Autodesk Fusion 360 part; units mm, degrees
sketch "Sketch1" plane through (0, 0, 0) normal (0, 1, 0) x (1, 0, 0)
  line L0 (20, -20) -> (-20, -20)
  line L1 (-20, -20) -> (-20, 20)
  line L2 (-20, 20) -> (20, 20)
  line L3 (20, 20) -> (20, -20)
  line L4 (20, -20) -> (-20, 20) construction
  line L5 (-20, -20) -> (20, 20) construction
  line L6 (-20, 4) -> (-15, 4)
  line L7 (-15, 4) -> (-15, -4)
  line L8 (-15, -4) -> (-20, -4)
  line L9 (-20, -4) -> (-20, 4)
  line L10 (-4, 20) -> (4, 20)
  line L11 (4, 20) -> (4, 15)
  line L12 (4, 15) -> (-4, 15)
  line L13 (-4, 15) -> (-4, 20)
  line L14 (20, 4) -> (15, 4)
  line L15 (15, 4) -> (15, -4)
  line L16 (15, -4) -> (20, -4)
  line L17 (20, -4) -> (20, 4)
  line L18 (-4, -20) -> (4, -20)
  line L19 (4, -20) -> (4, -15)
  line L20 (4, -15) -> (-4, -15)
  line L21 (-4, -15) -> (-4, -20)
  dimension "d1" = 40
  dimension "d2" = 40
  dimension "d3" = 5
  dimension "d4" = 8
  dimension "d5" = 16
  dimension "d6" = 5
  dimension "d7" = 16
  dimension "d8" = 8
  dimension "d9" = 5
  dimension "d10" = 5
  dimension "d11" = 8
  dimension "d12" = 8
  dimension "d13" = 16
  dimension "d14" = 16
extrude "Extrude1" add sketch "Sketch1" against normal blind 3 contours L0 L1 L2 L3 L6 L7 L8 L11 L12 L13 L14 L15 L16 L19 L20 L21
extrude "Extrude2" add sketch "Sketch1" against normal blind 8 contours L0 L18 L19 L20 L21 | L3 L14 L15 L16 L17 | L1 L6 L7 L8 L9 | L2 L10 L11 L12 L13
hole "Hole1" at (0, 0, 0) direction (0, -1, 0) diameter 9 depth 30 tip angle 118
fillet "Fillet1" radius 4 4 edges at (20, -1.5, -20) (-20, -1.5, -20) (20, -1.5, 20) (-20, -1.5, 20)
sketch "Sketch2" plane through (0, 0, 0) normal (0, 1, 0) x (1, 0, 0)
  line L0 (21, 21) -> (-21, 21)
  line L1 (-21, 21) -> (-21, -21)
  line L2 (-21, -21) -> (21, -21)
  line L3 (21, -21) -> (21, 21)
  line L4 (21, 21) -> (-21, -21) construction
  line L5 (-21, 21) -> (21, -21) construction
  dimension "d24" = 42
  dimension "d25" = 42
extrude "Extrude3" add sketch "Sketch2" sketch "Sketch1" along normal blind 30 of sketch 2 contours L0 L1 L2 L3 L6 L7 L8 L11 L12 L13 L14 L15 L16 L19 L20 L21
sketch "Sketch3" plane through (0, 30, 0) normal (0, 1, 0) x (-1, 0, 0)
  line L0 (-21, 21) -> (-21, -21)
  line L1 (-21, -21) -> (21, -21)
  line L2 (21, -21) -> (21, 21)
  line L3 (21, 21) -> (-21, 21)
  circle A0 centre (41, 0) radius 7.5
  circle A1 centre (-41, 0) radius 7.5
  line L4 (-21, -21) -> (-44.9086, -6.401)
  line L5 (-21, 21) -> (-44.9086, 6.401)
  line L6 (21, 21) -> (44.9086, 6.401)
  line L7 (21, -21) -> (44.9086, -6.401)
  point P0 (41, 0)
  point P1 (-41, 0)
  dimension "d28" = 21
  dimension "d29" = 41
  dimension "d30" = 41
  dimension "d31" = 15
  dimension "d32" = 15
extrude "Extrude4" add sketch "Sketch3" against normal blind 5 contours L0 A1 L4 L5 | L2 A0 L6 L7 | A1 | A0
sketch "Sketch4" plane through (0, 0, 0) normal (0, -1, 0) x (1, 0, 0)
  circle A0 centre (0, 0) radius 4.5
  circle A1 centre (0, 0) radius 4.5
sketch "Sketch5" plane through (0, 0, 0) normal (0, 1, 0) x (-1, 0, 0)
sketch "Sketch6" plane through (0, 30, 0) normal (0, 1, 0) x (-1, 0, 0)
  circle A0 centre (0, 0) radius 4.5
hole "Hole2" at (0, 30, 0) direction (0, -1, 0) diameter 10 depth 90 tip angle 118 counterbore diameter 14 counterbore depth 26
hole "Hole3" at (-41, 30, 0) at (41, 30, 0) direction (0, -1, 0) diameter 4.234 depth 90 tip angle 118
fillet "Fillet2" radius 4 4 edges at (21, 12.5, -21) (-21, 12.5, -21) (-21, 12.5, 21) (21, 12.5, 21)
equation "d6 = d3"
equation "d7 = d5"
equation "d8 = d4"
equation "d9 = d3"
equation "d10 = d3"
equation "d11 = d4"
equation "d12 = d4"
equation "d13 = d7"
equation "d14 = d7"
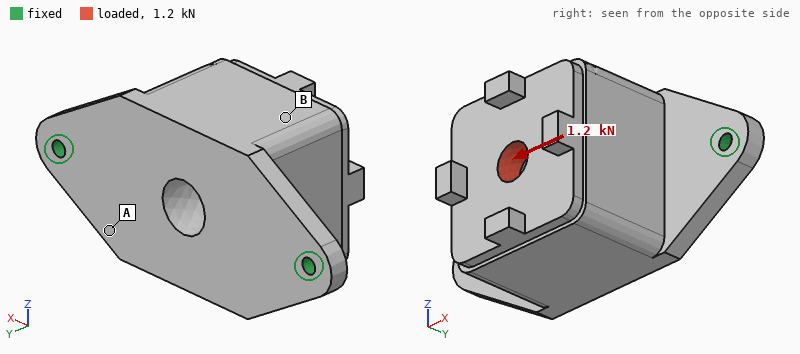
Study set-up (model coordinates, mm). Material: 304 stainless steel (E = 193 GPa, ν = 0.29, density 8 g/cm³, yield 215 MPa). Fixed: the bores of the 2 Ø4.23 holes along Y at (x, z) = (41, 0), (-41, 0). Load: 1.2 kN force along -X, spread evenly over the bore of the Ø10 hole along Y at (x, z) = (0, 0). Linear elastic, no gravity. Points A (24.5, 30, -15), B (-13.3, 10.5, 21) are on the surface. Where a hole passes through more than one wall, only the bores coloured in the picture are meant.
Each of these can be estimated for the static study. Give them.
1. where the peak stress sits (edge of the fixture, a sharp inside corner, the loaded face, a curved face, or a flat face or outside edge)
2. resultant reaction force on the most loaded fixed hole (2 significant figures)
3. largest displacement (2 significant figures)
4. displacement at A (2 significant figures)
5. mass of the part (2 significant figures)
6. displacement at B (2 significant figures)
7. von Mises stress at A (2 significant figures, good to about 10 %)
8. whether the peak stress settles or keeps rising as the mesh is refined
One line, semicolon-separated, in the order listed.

edge of the fixture; 780 N; 14 µm; 6.8 µm; 480 g; 7.6 µm; 23 MPa; keeps rising
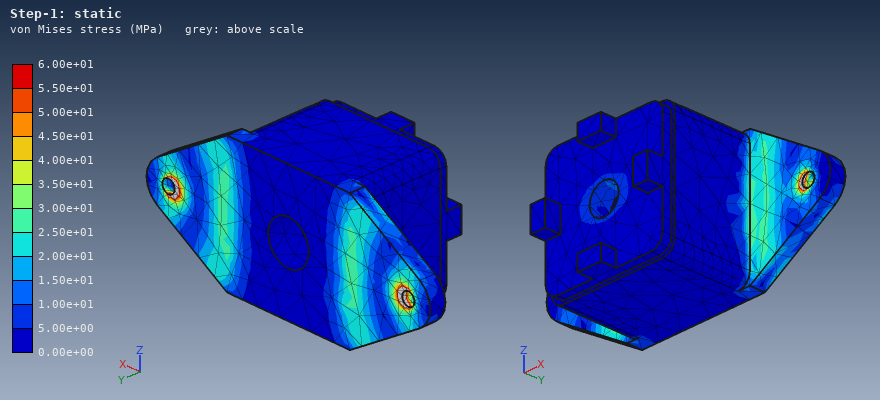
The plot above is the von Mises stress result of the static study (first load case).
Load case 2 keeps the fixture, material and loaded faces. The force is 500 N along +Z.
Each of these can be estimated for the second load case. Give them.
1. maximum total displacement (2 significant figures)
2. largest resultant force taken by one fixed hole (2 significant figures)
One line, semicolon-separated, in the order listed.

67 µm; 250 N
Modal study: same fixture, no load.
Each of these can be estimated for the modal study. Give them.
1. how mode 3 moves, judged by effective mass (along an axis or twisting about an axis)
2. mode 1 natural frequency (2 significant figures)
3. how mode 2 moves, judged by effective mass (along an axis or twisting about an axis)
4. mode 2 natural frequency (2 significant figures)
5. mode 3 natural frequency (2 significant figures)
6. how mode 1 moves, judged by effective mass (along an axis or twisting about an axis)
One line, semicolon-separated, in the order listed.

along X; 1000 Hz; along Y; 2300 Hz; 3400 Hz; along Z
